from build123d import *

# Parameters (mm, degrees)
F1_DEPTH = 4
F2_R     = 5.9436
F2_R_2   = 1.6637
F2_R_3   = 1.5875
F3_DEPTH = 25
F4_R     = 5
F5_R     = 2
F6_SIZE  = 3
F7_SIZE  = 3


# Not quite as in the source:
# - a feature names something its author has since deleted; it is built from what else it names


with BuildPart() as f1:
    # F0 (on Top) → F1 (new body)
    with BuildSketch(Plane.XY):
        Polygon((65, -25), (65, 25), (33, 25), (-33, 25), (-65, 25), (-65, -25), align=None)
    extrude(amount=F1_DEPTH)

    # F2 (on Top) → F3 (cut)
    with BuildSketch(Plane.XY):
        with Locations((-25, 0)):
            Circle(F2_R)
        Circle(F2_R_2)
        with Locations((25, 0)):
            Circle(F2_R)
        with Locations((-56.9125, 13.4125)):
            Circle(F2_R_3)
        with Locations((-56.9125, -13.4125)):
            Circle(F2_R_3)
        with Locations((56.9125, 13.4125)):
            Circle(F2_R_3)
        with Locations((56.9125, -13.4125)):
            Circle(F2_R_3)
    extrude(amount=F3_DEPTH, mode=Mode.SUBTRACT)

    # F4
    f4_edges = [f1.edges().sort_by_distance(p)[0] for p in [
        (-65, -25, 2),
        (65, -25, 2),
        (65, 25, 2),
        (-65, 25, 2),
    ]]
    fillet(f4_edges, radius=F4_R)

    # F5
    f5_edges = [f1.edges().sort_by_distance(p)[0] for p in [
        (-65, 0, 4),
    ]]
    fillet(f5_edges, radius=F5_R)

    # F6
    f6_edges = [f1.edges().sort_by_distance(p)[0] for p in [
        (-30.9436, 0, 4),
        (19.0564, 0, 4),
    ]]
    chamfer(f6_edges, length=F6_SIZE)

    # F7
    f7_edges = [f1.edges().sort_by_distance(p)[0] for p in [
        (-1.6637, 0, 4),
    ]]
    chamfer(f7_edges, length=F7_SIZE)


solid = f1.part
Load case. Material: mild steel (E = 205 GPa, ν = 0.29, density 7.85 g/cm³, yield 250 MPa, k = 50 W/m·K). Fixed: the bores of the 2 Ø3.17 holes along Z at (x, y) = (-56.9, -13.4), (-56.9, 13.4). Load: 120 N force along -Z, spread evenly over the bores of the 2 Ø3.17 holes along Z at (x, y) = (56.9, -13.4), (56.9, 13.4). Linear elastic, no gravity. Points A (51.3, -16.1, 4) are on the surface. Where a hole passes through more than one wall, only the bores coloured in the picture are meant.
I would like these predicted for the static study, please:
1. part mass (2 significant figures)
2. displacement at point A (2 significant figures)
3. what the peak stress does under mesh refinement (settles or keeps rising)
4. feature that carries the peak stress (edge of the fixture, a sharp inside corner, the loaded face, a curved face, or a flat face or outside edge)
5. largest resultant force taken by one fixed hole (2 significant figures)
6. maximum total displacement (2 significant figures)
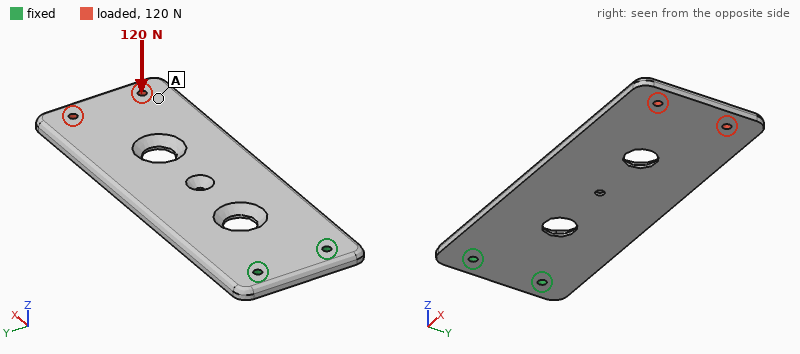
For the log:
190 g
1.2 mm
keeps rising
edge of the fixture
62 N
1.4 mm
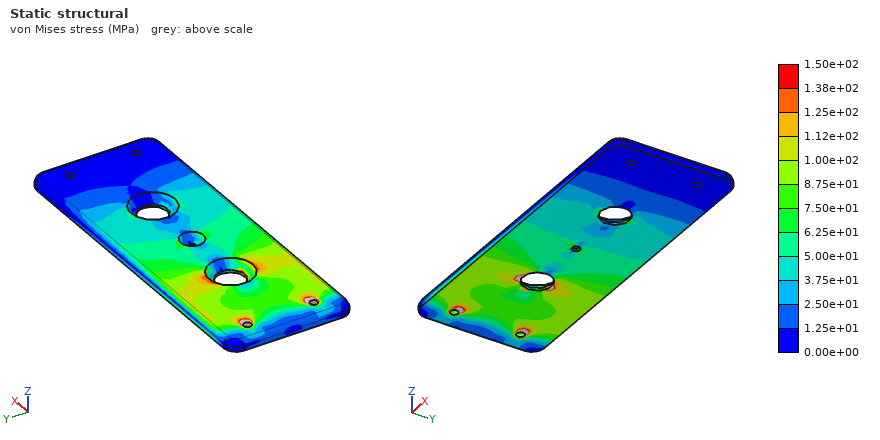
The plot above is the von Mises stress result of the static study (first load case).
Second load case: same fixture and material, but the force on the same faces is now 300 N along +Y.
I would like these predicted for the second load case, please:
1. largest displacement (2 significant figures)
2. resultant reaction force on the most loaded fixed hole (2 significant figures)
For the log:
31 µm
1.2 kN
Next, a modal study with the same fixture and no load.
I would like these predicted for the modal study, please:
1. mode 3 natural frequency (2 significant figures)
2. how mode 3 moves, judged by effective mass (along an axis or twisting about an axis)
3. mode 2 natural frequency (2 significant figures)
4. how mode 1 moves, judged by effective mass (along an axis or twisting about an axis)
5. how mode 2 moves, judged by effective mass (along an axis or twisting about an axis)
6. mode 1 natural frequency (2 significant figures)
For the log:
1300 Hz
along Z
1100 Hz
along Z
twisting about X
210 Hz
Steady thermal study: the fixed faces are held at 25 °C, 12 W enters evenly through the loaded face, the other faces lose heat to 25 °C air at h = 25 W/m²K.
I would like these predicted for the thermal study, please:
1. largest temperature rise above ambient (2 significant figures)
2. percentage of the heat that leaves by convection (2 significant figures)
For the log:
72 K
77 %
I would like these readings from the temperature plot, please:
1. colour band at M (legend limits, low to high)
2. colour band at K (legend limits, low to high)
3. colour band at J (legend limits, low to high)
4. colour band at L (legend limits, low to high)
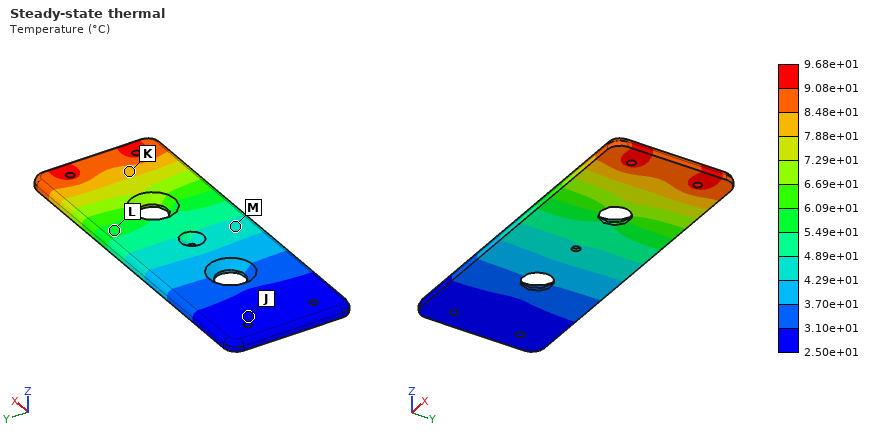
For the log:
4.29e+01 to 4.89e+01 °C
7.88e+01 to 8.48e+01 °C
2.50e+01 to 3.10e+01 °C
5.49e+01 to 6.09e+01 °C
